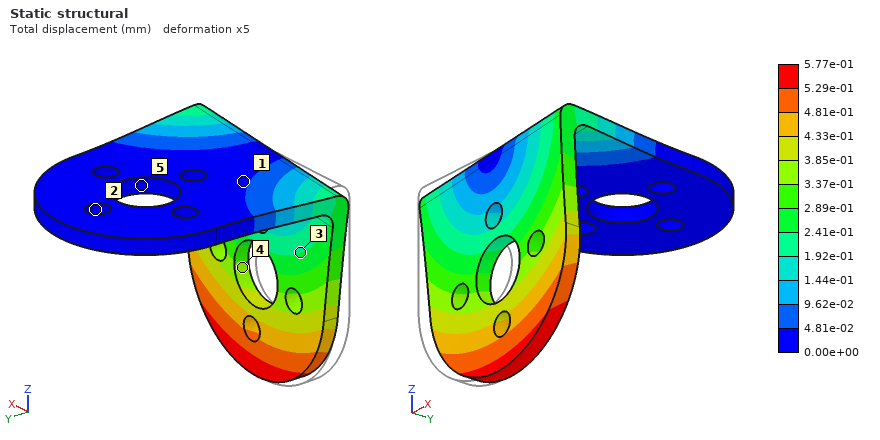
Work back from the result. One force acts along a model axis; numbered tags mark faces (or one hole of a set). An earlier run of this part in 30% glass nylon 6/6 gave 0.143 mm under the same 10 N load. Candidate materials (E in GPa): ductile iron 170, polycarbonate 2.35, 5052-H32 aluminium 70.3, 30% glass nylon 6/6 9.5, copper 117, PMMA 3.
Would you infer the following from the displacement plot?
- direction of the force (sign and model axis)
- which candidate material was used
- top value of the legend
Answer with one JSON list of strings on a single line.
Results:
["+X", "polycarbonate", "5.77e-01 mm"]
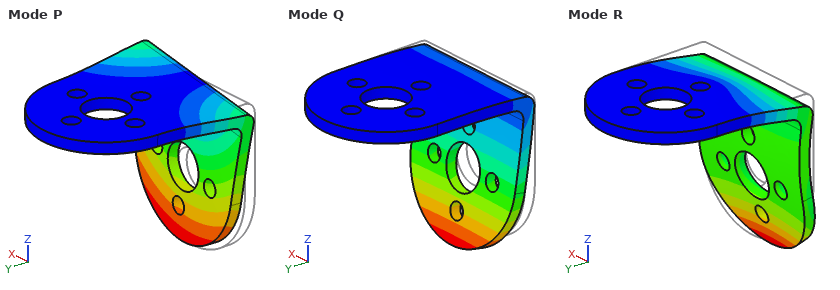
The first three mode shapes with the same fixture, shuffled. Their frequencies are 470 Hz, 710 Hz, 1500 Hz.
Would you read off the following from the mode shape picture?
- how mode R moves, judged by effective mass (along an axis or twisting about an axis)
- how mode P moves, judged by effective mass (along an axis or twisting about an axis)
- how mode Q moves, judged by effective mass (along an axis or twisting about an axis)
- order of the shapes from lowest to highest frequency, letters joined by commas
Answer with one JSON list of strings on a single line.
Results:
["along Z", "along X", "along Y", "Q, P, R"]
